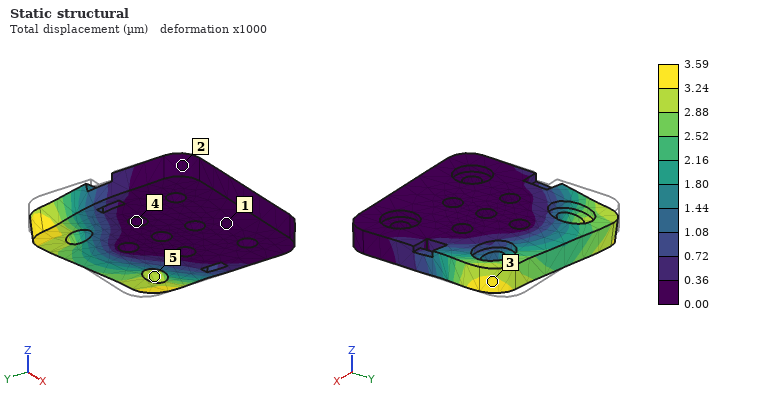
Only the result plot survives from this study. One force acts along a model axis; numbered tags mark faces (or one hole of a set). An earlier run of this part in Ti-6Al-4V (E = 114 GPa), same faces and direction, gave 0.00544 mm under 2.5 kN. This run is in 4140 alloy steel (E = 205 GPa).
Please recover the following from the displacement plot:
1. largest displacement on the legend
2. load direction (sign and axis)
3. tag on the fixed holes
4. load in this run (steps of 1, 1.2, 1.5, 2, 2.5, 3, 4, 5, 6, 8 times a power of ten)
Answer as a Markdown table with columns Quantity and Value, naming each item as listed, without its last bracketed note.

| Quantity | Value |
|---|---|
| largest displacement on the legend | 3.59 µm |
| load direction | +X |
| tag on the fixed holes | 4 |
| load in this run | 3 kN |
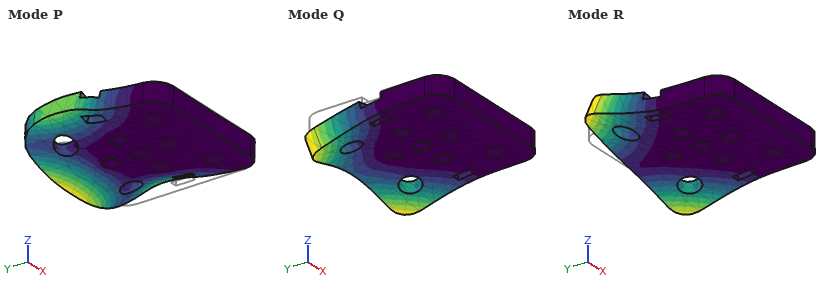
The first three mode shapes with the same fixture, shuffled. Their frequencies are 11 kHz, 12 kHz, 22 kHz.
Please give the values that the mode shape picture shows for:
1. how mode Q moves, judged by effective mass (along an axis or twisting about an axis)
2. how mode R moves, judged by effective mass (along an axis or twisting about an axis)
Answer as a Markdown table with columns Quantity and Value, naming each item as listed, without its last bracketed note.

| Quantity | Value |
|---|---|
| how mode Q moves, judged by effective mass | along Z |
| how mode R moves, judged by effective mass | twisting about Y |
